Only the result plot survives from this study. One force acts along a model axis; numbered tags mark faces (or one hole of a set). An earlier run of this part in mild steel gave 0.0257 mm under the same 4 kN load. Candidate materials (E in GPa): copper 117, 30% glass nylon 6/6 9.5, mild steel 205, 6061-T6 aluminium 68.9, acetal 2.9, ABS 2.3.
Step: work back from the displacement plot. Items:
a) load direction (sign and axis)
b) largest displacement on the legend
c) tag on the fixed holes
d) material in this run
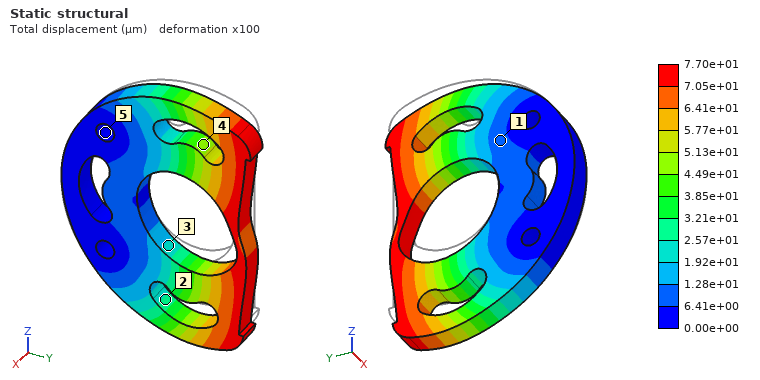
-Z
7.70e+01 µm
5
6061-T6 aluminium
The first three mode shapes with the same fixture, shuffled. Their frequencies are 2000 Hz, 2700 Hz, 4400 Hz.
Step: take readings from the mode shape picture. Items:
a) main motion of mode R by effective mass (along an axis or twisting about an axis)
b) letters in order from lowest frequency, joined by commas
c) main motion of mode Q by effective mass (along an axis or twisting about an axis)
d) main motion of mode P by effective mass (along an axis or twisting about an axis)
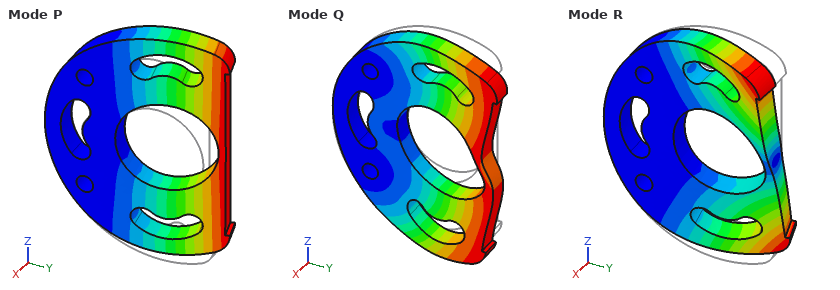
twisting about Y
P, R, Q
along Z
along X
